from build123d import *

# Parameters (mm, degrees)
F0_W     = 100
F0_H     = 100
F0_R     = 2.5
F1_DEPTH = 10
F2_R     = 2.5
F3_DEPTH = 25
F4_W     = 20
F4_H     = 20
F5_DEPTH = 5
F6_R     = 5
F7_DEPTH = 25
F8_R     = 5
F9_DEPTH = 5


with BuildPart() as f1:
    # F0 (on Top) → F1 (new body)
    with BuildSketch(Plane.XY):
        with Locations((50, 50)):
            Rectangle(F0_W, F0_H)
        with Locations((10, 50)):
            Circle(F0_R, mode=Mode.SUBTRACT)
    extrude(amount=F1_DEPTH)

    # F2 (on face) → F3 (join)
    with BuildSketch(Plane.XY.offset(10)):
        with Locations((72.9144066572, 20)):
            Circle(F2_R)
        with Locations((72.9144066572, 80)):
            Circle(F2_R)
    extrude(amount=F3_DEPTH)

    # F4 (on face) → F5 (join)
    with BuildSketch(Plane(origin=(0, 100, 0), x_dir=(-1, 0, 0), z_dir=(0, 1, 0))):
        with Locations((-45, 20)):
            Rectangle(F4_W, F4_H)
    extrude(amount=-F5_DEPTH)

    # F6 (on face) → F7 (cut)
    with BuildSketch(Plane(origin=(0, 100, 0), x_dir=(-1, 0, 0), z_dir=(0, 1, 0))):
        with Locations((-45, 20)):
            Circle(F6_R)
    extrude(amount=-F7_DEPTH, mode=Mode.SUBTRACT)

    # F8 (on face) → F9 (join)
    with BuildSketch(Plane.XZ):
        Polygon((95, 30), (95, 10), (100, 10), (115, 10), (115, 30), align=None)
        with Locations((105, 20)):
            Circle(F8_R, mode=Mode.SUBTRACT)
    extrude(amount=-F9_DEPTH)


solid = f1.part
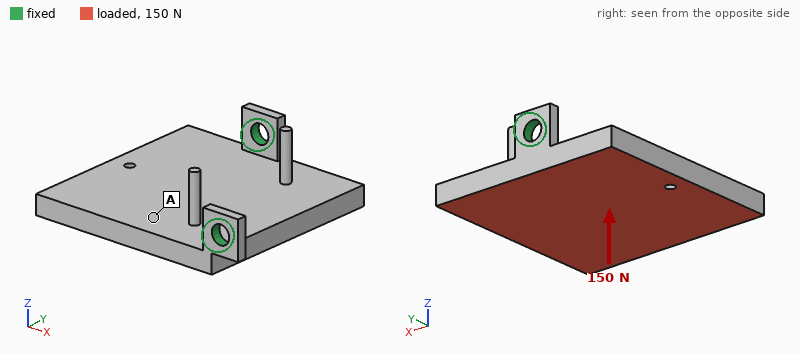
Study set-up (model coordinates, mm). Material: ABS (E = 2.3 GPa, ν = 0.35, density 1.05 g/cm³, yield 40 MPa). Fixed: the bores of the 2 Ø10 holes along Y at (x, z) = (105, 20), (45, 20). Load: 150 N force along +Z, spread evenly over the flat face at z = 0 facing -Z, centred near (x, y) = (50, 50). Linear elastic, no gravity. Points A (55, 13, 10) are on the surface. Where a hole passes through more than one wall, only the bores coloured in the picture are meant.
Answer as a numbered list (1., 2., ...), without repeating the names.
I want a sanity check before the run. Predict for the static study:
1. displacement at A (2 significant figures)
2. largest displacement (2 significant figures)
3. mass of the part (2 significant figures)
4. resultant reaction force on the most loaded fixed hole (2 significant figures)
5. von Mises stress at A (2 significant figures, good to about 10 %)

1. 0.66 mm
2. 1.7 mm
3. 110 g
4. 110 N
5. 1.5 MPa
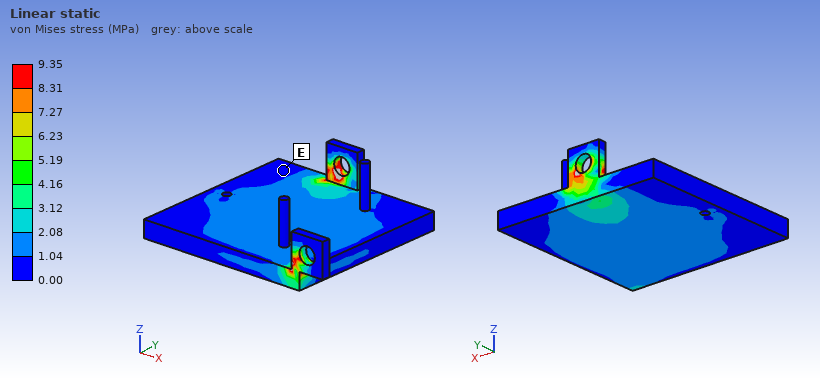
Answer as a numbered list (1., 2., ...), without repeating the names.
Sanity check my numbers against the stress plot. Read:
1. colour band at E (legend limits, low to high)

1. 0.00 to 1.04 MPa
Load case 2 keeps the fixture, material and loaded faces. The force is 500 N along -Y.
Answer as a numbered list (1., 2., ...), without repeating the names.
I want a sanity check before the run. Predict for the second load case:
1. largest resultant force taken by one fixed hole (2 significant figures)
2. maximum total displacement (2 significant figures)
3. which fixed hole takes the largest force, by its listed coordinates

1. 360 N
2. 1.5 mm
3. (45, 20)
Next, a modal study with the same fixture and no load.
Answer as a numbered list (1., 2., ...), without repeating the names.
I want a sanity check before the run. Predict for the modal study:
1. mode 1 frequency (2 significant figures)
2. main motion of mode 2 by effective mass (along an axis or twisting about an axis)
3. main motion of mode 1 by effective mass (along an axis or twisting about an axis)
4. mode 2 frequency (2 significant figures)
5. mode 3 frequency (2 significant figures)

1. 190 Hz
2. along Z
3. along Z
4. 650 Hz
5. 840 Hz
